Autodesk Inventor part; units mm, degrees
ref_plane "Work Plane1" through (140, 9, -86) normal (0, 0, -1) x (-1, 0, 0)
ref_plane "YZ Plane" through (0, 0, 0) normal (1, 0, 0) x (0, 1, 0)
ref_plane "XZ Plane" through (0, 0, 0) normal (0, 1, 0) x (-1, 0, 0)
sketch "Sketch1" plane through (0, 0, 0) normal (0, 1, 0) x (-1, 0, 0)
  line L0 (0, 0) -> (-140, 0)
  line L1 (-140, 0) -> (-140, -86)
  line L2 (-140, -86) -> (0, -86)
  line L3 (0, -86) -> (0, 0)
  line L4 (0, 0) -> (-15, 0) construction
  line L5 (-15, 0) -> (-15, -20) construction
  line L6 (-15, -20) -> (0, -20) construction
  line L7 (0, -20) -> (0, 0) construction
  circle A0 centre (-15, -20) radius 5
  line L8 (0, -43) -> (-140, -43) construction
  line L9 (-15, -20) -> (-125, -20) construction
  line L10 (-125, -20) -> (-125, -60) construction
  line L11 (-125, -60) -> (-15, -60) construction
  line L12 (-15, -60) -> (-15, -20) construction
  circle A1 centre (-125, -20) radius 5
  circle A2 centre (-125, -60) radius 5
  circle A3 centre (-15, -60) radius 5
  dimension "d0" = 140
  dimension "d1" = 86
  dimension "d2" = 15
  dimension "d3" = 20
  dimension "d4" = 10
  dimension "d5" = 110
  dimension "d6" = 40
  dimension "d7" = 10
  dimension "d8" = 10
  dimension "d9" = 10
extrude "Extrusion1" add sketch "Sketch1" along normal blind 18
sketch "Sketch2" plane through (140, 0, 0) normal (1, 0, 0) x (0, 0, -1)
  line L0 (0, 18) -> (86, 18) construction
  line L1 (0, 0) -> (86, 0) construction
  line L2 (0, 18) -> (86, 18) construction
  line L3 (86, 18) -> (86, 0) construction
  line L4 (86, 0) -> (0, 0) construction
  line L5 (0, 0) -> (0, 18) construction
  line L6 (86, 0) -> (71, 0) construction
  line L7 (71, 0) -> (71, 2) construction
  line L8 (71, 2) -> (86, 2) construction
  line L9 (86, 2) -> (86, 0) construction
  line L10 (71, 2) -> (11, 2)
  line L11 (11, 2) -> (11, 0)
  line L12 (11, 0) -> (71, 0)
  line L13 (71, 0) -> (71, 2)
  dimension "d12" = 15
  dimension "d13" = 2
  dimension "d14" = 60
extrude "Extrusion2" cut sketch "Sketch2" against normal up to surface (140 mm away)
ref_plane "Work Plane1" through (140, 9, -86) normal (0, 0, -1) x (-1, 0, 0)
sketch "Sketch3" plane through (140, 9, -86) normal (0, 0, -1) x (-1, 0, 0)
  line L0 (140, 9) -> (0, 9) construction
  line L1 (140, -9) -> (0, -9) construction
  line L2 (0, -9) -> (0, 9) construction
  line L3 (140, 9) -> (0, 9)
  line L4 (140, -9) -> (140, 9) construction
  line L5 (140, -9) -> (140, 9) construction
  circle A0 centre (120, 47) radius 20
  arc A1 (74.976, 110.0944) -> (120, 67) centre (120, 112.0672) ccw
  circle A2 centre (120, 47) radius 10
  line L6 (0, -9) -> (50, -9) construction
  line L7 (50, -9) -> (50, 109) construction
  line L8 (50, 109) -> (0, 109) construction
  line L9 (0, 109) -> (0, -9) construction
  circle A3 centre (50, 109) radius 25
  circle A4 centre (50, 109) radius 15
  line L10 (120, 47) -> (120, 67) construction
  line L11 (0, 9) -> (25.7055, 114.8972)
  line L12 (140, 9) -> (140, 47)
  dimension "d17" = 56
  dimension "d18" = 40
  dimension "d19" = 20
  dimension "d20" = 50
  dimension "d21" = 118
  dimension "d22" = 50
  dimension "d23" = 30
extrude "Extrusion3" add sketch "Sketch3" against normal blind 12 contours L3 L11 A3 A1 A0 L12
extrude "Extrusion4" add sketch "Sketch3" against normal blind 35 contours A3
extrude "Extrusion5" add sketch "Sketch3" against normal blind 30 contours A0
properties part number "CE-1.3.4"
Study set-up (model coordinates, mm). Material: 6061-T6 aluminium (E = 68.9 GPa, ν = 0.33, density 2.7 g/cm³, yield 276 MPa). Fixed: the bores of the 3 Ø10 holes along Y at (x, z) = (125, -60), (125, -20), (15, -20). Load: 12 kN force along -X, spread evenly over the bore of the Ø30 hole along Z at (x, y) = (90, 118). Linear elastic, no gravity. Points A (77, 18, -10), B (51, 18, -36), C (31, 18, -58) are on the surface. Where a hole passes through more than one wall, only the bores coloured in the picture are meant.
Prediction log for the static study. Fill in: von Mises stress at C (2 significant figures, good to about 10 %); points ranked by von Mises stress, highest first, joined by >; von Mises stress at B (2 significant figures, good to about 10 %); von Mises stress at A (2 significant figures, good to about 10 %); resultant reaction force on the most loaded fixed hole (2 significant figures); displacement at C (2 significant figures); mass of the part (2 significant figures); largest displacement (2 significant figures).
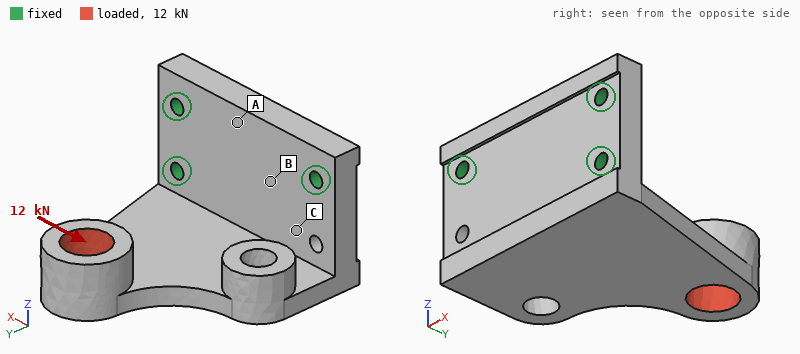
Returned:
95 MPa
C > B > A
61 MPa
24 MPa
11 kN
0.22 mm
990 g
1.2 mm
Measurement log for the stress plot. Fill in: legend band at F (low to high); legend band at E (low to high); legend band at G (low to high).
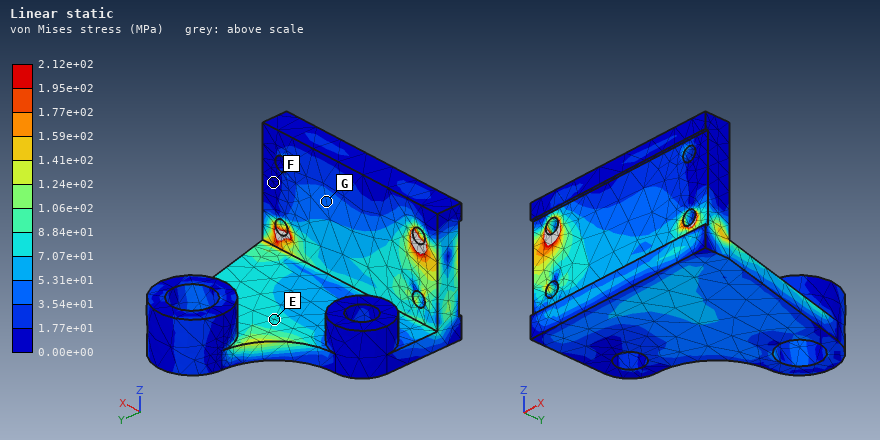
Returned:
0.00e+00 to 1.77e+01 MPa
7.07e+01 to 8.84e+01 MPa
3.54e+01 to 5.31e+01 MPa
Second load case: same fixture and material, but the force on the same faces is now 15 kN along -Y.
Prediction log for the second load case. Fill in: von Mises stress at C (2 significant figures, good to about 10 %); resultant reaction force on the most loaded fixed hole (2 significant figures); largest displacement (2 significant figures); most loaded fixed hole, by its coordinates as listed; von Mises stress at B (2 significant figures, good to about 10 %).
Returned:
20 MPa
12 kN
1.2 mm
(125, -60)
15 MPa
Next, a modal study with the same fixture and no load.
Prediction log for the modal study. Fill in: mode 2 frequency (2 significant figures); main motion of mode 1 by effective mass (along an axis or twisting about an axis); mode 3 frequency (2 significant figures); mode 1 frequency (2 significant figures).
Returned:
1200 Hz
along Z
2300 Hz
590 Hz
